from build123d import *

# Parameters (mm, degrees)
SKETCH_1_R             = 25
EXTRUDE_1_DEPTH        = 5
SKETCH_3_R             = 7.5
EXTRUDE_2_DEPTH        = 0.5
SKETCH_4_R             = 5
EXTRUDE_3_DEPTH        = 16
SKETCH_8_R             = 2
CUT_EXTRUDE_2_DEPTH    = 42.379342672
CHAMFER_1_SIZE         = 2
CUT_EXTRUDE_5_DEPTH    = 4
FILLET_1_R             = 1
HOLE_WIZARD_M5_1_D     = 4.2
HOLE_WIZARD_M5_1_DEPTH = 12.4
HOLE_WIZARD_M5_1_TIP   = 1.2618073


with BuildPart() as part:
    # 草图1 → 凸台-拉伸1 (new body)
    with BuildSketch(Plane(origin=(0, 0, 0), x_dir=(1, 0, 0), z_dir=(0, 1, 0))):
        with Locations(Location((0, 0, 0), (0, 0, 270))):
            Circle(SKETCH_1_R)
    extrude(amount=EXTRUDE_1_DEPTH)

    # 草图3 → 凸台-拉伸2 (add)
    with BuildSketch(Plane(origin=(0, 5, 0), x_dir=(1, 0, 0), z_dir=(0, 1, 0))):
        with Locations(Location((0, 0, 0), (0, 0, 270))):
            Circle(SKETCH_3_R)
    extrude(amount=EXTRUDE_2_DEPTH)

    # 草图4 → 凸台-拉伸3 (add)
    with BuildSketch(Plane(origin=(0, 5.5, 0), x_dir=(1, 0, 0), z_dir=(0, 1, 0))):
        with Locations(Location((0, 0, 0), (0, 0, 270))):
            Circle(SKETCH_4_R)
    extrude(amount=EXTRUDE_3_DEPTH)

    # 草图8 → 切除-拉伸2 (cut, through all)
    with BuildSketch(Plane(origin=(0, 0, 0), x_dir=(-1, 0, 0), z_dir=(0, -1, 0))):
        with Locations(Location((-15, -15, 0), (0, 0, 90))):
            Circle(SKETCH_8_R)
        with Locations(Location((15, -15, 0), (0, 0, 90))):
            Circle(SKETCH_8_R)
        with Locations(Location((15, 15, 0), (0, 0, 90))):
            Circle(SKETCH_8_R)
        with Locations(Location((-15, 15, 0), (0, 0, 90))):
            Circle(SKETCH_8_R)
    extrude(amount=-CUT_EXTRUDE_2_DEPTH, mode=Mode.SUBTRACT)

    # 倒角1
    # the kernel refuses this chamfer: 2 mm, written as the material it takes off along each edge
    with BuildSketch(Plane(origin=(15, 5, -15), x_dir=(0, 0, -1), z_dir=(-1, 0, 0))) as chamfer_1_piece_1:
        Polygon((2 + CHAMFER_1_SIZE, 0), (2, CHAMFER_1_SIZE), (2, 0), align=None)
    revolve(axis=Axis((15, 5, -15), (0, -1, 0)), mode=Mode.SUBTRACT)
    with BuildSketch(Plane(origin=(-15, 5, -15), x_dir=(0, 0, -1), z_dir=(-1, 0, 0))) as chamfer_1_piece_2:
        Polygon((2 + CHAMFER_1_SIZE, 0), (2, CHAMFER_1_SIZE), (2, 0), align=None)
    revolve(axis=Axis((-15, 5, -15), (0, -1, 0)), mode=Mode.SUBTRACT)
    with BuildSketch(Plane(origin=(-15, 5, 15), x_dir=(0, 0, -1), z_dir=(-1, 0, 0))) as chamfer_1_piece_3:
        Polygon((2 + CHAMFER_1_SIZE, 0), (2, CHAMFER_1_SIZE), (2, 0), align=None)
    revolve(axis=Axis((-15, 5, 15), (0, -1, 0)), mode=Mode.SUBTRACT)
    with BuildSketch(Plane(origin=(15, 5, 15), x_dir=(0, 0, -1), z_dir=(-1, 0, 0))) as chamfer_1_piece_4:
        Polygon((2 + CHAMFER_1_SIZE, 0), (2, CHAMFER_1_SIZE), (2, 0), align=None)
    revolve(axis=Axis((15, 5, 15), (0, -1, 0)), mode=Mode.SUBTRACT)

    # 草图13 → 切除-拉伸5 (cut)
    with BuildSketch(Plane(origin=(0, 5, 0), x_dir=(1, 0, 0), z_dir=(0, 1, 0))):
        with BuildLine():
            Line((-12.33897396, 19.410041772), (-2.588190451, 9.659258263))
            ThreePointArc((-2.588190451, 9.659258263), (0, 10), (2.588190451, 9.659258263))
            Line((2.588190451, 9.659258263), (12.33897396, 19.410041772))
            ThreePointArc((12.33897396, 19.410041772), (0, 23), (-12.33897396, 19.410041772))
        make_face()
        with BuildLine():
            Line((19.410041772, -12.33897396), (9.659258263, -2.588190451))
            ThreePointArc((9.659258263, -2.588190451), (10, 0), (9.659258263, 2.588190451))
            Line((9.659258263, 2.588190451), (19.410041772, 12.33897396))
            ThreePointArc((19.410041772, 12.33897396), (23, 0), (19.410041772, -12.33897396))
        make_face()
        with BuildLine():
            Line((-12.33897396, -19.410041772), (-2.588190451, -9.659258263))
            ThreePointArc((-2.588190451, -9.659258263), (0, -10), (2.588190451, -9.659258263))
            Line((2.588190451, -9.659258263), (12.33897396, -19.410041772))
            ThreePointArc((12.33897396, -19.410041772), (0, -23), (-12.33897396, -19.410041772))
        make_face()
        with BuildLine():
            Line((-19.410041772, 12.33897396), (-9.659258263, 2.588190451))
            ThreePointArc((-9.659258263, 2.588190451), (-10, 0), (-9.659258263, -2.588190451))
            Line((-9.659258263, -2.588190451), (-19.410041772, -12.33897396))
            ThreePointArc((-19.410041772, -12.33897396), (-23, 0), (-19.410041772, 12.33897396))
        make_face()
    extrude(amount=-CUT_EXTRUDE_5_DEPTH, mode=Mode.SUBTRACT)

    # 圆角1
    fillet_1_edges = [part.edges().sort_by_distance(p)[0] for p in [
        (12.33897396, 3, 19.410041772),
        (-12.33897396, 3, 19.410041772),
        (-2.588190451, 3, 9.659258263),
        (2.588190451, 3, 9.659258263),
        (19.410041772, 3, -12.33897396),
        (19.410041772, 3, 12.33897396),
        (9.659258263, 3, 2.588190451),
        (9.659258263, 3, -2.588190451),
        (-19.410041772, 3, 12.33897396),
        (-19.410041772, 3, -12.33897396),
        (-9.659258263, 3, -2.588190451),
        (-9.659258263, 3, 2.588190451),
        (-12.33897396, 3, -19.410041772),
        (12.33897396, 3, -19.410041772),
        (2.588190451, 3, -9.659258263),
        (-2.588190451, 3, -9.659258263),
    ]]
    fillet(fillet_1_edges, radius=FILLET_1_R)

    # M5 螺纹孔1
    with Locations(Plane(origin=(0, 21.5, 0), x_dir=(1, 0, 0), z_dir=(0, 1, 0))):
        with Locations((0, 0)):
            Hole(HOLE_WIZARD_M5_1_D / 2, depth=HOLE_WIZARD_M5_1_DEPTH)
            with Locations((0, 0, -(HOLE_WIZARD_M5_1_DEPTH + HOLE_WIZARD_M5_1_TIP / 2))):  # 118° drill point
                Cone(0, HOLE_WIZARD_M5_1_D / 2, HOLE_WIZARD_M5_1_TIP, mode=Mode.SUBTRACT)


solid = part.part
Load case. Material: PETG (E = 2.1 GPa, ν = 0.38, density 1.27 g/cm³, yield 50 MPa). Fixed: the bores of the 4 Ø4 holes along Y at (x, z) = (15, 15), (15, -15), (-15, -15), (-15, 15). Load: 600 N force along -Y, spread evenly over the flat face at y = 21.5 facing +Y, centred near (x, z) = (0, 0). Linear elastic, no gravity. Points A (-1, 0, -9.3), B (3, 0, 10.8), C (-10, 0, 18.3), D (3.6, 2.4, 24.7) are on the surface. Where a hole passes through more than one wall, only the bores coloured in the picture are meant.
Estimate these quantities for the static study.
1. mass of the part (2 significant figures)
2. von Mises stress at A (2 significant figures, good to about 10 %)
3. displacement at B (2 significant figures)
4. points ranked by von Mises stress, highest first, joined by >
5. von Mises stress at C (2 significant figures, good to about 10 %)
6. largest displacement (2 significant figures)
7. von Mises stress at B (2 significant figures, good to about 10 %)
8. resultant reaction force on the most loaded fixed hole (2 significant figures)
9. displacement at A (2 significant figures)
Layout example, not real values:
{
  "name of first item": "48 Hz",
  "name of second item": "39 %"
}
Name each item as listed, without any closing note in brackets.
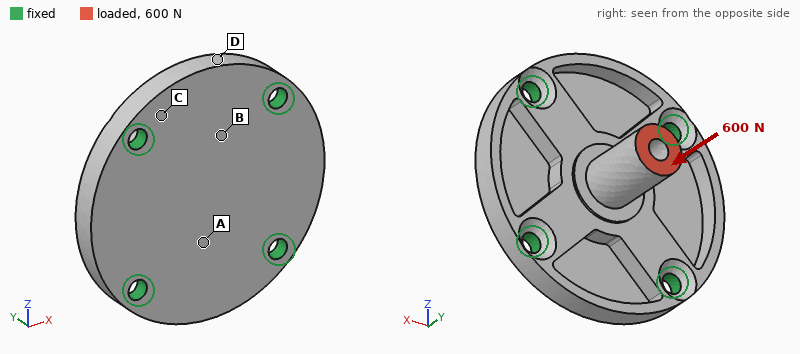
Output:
{
  "mass of the part": "9.3 g",
  "von Mises stress at A": "17 MPa",
  "displacement at B": "0.24 mm",
  "points ranked by von Mises stress, highest first, joined by >": "A > B > C > D",
  "von Mises stress at C": "7.4 MPa",
  "largest displacement": "0.39 mm",
  "von Mises stress at B": "12 MPa",
  "resultant reaction force on the most loaded fixed hole": "170 N",
  "displacement at A": "0.28 mm"
}
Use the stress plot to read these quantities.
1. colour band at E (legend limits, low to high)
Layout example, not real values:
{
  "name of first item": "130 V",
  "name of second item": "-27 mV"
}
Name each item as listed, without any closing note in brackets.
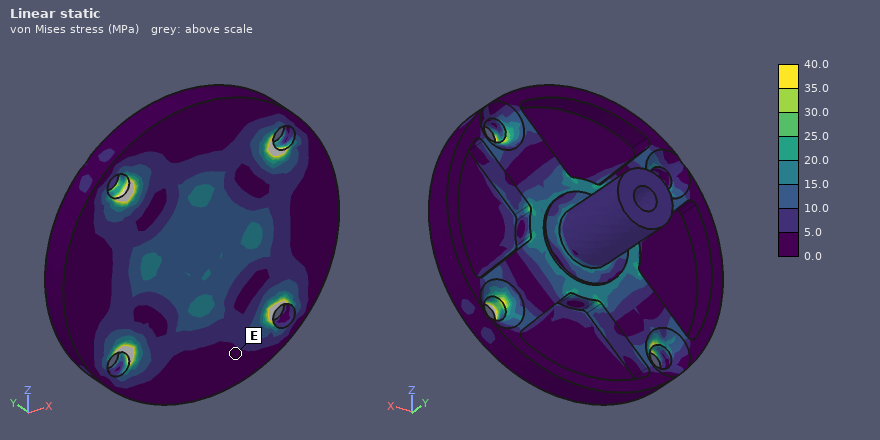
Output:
{
  "colour band at E": "0.0 to 5.0 MPa"
}
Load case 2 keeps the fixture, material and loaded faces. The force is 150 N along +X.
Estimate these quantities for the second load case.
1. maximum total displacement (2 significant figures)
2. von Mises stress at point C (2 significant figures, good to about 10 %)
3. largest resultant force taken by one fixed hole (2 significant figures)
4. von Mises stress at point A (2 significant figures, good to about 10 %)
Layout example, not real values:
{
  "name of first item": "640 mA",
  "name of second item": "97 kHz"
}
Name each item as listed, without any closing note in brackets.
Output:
{
  "maximum total displacement": "0.60 mm",
  "von Mises stress at point C": "1.4 MPa",
  "largest resultant force taken by one fixed hole": "74 N",
  "von Mises stress at point A": "4.9 MPa"
}
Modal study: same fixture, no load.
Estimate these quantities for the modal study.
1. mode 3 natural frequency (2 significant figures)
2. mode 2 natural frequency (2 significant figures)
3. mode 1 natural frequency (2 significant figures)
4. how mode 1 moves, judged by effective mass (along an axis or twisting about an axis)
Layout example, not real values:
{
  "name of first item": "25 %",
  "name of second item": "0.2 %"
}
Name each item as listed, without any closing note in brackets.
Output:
{
  "mode 3 natural frequency": "3700 Hz",
  "mode 2 natural frequency": "3700 Hz",
  "mode 1 natural frequency": "3400 Hz",
  "how mode 1 moves, judged by effective mass": "along Y"
}
